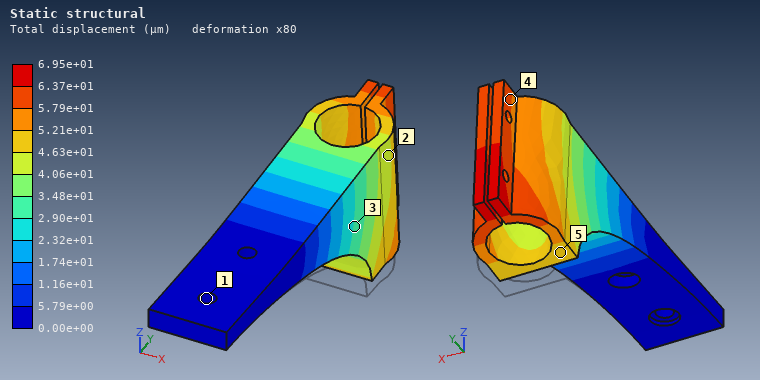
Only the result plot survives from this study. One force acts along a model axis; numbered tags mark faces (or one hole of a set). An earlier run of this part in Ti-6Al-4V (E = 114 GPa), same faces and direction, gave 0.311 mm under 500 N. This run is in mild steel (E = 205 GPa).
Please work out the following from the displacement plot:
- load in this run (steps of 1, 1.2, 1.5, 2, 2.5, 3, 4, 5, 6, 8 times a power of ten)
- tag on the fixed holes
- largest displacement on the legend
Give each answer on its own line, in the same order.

200 N
1
6.95e+01 µm
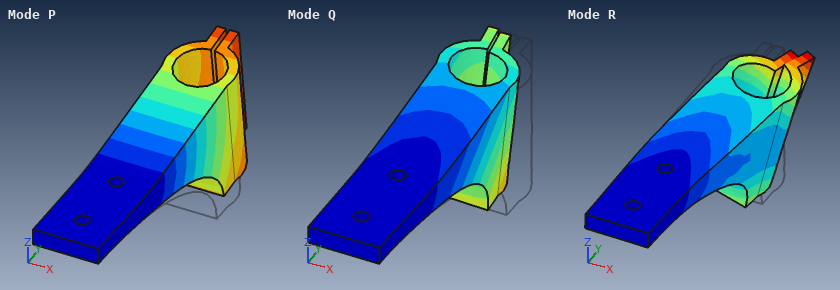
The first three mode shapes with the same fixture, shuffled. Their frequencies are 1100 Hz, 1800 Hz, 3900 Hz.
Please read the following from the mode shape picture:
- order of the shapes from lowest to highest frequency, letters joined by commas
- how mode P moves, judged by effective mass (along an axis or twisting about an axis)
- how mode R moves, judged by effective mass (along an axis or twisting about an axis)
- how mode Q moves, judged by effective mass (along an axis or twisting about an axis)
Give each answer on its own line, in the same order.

P, Q, R
along Z
twisting about Y
along X
